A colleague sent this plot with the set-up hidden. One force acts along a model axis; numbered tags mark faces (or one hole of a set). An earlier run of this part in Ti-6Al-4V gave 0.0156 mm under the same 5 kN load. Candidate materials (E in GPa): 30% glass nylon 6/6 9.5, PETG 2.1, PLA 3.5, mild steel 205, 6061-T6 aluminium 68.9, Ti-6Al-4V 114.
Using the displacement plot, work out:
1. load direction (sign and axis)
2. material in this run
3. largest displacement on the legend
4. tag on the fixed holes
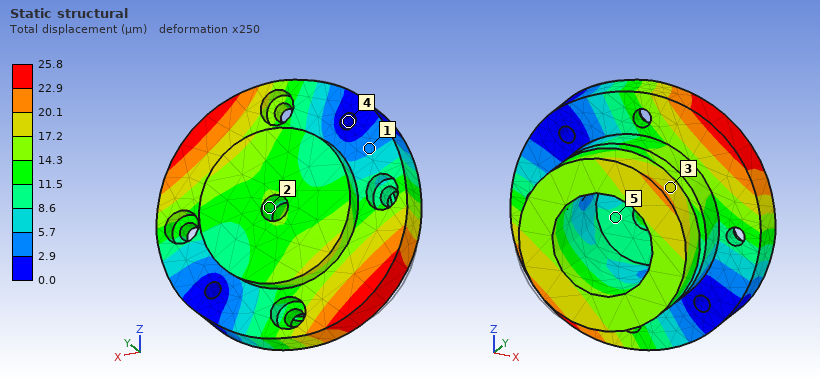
-Z
6061-T6 aluminium
25.8 µm
4
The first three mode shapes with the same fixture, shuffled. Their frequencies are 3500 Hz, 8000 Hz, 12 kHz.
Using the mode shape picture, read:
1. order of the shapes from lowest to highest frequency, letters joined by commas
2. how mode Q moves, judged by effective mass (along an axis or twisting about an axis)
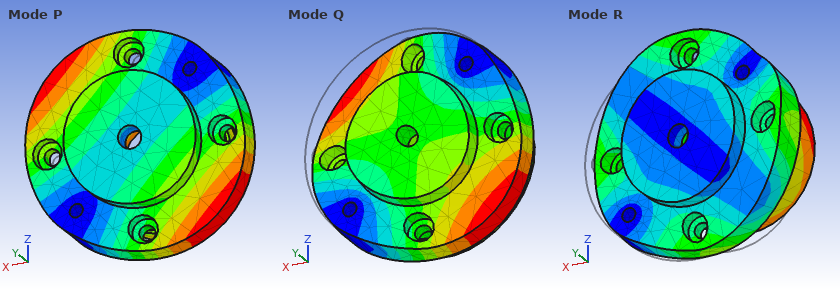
P, Q, R
along Y
